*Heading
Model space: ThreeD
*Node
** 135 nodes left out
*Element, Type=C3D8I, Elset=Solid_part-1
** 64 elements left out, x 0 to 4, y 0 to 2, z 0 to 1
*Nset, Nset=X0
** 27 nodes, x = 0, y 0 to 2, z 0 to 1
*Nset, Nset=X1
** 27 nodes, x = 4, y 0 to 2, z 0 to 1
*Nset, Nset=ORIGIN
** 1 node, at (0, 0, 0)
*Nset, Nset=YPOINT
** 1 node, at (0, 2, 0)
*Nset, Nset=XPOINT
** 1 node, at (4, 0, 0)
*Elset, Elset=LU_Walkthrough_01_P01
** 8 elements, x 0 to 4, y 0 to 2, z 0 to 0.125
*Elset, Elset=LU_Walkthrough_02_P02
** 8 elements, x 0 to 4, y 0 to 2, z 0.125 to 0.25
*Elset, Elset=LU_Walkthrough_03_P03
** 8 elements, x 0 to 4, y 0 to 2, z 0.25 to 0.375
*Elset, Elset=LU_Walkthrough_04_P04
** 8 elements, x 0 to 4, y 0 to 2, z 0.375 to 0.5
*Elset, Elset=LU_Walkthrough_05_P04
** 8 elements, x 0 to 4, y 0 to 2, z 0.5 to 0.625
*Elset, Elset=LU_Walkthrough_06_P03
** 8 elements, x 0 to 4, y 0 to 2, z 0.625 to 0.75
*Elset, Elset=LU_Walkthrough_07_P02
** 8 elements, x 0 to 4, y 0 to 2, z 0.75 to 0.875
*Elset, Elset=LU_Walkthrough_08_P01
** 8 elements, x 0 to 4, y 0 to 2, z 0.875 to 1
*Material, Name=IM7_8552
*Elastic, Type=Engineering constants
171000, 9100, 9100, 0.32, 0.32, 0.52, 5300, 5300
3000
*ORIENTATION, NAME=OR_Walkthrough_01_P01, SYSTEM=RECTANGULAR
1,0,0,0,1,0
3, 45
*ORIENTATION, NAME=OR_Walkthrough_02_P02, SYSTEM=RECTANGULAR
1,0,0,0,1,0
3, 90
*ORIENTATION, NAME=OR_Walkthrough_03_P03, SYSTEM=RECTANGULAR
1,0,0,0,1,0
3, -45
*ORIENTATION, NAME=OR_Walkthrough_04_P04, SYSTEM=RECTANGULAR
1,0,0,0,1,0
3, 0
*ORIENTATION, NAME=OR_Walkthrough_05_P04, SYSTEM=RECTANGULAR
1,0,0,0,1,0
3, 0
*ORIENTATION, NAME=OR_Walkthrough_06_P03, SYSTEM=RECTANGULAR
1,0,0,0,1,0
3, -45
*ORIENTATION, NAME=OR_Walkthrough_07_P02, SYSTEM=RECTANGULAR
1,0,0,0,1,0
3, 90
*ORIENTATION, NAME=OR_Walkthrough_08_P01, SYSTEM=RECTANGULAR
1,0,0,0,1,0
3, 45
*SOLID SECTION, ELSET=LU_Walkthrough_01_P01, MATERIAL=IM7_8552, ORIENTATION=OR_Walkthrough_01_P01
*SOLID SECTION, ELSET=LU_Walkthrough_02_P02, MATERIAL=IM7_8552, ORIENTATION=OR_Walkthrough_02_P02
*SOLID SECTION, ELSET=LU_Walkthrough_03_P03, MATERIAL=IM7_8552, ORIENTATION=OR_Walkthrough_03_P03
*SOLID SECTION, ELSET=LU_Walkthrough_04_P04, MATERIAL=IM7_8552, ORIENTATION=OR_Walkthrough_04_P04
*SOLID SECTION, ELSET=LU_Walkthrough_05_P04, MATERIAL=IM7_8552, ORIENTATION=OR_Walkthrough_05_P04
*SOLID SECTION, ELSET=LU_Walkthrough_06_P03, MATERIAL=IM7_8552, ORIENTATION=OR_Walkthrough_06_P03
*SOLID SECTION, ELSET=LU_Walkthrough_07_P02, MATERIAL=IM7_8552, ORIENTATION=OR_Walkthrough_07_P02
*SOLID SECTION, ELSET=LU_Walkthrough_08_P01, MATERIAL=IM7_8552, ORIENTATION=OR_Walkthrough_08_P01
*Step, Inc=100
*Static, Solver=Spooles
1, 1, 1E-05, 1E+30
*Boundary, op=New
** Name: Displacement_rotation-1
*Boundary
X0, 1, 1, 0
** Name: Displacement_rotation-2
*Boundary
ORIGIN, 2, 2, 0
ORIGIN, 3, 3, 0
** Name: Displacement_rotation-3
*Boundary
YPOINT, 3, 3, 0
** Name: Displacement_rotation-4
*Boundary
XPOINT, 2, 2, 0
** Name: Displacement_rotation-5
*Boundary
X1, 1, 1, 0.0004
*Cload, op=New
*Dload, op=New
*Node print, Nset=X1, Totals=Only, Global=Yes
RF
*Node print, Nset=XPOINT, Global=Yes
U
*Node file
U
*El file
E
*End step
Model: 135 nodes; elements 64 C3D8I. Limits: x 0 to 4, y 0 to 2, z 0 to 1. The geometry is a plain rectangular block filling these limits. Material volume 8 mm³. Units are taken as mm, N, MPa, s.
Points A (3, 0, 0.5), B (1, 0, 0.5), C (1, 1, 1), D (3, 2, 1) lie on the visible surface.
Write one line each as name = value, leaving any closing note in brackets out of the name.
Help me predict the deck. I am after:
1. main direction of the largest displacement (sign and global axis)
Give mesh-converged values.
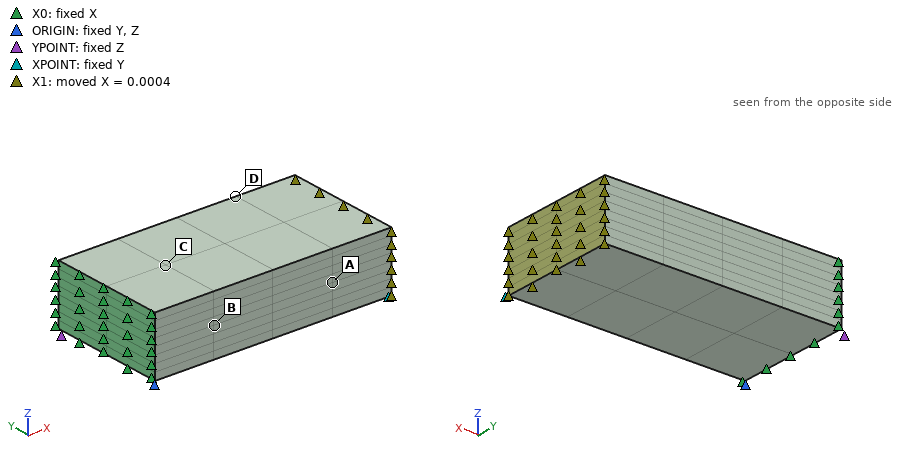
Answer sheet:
main direction of the largest displacement = +X
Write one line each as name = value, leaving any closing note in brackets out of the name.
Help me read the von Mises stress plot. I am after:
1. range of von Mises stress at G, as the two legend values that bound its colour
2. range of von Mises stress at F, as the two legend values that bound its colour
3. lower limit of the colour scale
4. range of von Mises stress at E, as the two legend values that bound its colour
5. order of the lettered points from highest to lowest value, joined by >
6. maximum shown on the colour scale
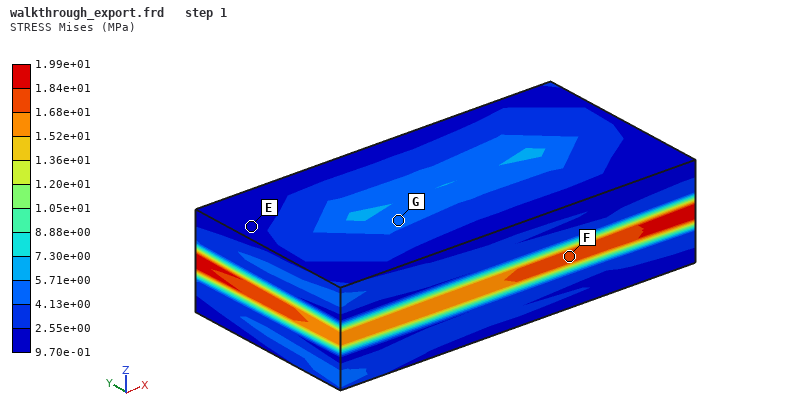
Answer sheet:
range of von Mises stress at G, as the two legend values that bound its colour = 4.13e+00 to 5.71e+00 MPa
range of von Mises stress at F, as the two legend values that bound its colour = 1.68e+01 to 1.84e+01 MPa
lower limit of the colour scale = 9.70e-01 MPa
range of von Mises stress at E, as the two legend values that bound its colour = 9.70e-01 to 2.55e+00 MPa
order of the lettered points from highest to lowest value, joined by > = F > G > E
maximum shown on the colour scale = 1.99e+01 MPa
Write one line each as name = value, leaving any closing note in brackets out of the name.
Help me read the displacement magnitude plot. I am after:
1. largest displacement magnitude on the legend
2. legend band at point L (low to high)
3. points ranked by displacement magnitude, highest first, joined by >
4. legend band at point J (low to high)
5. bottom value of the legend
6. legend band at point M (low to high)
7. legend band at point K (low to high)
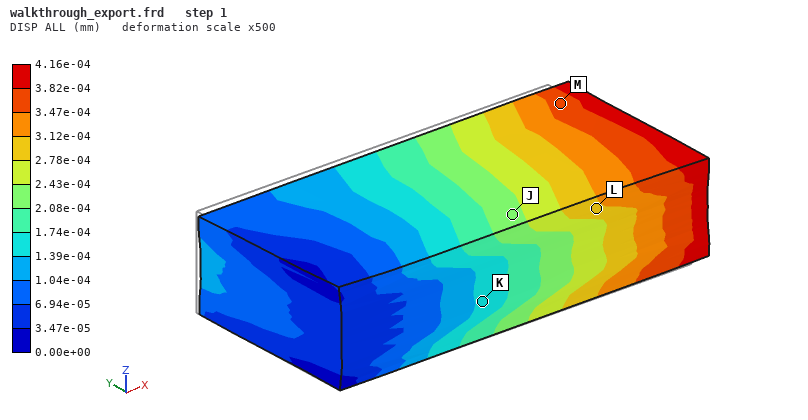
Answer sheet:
largest displacement magnitude on the legend = 4.16e-04 mm
legend band at point L = 2.78e-04 to 3.12e-04 mm
points ranked by displacement magnitude, highest first, joined by > = M > L > J > K
legend band at point J = 2.08e-04 to 2.43e-04 mm
bottom value of the legend = 0.00e+00 mm
legend band at point M = 3.47e-04 to 3.82e-04 mm
legend band at point K = 1.39e-04 to 1.74e-04 mm
